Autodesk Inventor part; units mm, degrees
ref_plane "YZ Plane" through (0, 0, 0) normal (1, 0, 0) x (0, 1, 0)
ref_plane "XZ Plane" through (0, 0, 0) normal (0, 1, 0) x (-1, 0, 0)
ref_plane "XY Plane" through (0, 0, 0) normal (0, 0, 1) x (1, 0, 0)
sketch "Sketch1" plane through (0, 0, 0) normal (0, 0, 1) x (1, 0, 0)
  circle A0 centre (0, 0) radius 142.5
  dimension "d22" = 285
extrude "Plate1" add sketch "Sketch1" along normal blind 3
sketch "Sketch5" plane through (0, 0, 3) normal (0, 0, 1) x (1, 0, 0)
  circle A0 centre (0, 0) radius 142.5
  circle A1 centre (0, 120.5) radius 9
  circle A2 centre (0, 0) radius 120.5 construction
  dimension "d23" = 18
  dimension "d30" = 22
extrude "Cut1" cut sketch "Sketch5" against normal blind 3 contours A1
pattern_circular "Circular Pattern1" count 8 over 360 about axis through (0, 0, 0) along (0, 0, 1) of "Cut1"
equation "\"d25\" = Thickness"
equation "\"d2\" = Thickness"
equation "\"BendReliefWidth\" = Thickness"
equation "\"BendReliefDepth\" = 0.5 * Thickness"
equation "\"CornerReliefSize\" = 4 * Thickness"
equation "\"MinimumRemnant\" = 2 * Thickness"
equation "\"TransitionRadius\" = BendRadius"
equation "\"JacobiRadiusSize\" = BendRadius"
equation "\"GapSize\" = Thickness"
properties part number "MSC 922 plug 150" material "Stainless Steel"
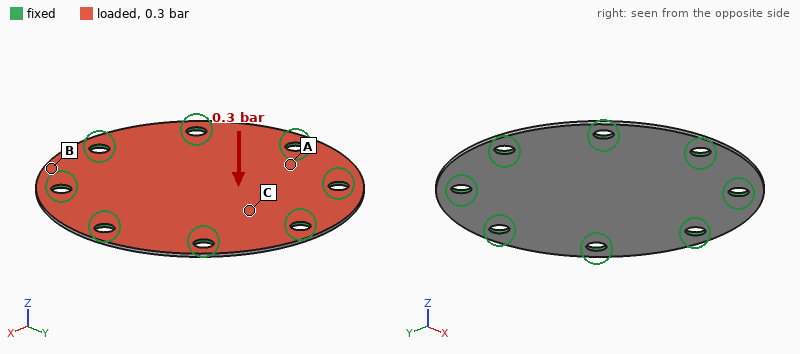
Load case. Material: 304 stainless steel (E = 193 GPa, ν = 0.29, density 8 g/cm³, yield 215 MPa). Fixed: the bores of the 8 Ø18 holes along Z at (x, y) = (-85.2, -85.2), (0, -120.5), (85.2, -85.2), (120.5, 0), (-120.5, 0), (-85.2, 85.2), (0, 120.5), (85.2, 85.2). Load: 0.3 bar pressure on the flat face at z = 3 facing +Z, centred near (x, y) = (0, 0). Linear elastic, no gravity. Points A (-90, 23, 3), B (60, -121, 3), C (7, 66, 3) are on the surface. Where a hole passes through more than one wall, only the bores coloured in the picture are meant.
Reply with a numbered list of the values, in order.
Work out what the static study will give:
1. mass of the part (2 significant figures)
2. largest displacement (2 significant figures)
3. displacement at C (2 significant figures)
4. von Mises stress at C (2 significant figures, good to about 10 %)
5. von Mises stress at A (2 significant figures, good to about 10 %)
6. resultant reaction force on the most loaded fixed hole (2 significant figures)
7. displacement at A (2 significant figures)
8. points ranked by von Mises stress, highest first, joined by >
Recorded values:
1. 1.5 kg
2. 0.19 mm
3. 0.092 mm
4. 9.7 MPa
5. 17 MPa
6. 230 N
7. 0.034 mm
8. A > C > B
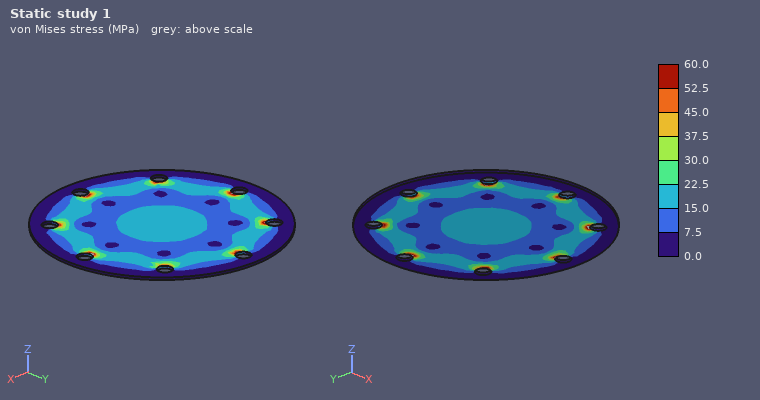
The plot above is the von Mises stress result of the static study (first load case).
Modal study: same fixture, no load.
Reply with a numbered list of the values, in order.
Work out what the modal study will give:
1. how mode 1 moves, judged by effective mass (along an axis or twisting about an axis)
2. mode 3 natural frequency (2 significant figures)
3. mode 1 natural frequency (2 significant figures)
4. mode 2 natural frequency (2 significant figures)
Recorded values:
1. along Z
2. 1000 Hz
3. 510 Hz
4. 1000 Hz
